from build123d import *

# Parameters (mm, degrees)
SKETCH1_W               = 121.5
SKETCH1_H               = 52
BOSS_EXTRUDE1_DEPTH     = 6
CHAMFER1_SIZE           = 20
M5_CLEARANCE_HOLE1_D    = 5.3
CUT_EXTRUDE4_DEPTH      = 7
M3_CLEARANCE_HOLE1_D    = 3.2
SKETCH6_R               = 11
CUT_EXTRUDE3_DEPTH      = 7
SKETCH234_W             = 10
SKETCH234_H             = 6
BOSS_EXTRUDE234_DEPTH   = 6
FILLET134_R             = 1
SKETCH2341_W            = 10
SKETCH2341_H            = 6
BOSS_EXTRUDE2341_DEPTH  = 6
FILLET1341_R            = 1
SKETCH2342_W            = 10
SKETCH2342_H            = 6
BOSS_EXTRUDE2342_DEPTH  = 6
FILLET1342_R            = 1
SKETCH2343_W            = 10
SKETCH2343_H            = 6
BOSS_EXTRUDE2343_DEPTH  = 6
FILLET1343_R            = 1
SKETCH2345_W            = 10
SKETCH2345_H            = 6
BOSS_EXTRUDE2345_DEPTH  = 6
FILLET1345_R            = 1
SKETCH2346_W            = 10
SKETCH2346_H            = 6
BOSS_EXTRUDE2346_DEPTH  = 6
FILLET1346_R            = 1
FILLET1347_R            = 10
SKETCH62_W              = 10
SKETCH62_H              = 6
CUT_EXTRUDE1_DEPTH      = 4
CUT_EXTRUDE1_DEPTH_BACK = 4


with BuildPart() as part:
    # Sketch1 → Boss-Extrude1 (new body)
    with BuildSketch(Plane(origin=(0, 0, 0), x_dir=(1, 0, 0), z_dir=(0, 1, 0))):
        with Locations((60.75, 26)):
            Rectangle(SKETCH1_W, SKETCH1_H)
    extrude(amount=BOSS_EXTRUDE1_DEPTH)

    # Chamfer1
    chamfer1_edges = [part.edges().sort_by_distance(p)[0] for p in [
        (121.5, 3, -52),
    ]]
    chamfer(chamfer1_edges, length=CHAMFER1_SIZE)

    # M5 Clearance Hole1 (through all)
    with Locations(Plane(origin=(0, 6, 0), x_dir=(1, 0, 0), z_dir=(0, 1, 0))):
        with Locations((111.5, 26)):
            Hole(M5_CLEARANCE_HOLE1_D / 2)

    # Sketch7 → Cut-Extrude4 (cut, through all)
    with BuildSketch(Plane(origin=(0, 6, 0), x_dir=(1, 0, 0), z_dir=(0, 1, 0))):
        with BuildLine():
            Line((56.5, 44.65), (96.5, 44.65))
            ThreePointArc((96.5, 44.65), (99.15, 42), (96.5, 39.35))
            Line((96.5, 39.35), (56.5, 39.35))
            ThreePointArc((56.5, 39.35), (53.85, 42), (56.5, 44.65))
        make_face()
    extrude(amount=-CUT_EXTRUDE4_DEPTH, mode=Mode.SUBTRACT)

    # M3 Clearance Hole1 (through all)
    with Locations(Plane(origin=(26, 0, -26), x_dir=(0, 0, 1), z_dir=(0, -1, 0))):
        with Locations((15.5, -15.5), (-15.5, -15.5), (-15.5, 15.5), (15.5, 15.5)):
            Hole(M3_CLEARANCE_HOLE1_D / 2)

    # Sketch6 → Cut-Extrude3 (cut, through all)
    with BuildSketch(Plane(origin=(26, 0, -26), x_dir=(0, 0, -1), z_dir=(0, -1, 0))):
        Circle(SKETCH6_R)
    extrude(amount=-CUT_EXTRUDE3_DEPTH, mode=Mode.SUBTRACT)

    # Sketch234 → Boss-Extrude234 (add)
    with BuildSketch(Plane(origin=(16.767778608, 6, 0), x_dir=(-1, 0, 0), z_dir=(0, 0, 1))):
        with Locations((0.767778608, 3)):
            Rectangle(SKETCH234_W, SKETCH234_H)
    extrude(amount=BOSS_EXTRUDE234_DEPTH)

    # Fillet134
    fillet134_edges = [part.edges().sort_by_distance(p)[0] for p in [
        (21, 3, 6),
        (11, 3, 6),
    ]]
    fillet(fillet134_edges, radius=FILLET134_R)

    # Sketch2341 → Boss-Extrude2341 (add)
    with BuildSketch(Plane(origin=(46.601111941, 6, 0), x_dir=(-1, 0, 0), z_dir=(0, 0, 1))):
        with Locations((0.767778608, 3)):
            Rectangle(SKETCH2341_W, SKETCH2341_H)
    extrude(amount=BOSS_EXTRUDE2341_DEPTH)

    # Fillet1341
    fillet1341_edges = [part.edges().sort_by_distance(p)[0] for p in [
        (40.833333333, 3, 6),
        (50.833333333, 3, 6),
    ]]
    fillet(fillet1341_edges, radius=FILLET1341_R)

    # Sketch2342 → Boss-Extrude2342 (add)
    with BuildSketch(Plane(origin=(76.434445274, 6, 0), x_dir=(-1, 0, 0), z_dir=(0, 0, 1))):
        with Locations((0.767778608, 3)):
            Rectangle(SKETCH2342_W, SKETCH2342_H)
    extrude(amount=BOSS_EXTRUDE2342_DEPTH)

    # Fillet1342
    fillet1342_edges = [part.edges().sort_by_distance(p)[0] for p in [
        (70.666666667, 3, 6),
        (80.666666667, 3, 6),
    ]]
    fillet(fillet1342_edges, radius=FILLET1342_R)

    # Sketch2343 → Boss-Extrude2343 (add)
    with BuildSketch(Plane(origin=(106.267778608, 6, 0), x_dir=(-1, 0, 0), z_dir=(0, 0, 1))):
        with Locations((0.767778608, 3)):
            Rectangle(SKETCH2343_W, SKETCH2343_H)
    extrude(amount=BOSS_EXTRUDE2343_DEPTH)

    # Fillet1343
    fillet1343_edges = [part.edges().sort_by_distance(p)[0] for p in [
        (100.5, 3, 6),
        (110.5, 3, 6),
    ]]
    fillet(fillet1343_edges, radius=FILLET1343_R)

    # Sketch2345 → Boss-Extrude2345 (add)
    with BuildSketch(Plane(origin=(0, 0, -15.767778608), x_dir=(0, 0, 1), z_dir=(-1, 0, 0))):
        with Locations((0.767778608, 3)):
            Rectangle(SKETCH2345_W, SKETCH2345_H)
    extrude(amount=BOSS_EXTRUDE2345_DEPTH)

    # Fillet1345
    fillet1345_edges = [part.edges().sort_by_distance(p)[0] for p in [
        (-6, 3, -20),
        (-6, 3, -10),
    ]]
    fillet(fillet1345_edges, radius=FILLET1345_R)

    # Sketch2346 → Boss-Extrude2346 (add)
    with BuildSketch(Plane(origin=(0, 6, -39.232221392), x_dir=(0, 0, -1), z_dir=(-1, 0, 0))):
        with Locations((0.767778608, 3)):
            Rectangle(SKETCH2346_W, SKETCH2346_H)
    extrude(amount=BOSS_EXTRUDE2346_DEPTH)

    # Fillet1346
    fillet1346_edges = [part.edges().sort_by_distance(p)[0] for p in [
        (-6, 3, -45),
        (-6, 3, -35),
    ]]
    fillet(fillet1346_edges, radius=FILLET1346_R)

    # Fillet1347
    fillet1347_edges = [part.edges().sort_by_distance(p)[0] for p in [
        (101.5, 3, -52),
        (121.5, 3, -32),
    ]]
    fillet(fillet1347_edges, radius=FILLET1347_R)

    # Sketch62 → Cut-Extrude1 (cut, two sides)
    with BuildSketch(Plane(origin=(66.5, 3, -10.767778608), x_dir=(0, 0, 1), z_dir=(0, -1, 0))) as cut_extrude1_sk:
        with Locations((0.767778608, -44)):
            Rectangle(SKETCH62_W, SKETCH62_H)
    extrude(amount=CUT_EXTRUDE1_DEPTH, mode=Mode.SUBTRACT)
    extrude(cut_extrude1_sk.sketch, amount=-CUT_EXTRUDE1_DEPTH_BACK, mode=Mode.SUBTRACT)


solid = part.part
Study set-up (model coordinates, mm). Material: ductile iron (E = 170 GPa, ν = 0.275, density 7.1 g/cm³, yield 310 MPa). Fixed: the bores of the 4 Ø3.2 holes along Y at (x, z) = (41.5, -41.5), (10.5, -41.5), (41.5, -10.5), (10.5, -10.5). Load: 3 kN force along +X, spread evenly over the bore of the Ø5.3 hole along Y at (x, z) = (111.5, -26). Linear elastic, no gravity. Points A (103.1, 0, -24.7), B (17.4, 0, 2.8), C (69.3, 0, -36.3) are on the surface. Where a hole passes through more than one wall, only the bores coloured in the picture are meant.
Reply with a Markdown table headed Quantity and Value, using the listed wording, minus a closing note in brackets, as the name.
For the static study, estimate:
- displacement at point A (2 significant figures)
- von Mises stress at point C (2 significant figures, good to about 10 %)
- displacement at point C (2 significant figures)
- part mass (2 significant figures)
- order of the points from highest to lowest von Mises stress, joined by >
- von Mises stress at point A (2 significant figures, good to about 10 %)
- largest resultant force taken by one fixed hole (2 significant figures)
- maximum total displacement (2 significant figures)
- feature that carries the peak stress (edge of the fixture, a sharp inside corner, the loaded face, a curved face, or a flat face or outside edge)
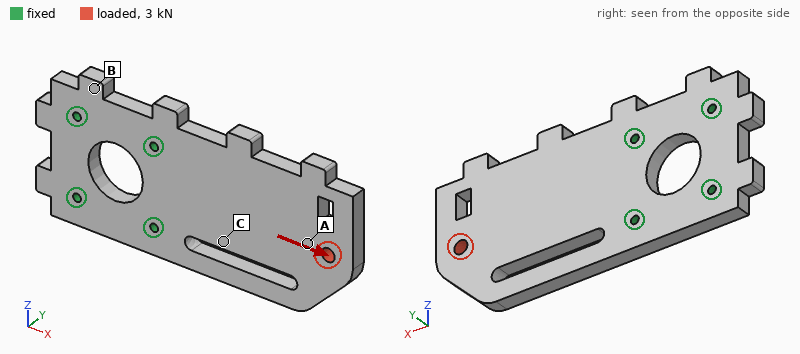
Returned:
| Quantity | Value |
|---|---|
| displacement at point A | 6.0 µm |
| von Mises stress at point C | 15 MPa |
| displacement at point C | 2.9 µm |
| part mass | 240 g |
| order of the points from highest to lowest von Mises stress, joined by > | A > C > B |
| von Mises stress at point A | 25 MPa |
| largest resultant force taken by one fixed hole | 1.4 kN |
| maximum total displacement | 8.0 µm |
| feature that carries the peak stress | the loaded face |
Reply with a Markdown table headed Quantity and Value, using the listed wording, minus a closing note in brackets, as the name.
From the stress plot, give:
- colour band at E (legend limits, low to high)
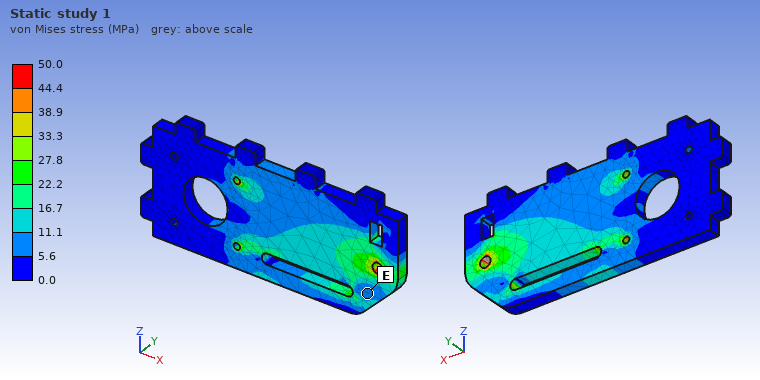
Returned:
| Quantity | Value |
|---|---|
| colour band at E | 5.6 to 11.1 MPa |
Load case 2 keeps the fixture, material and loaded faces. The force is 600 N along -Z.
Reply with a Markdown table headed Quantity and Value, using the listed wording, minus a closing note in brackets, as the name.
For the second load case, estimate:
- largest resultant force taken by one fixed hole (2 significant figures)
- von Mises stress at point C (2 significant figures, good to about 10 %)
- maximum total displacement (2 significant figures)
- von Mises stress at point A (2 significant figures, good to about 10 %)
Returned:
| Quantity | Value |
|---|---|
| largest resultant force taken by one fixed hole | 1.1 kN |
| von Mises stress at point C | 8.1 MPa |
| maximum total displacement | 15 µm |
| von Mises stress at point A | 4.4 MPa |
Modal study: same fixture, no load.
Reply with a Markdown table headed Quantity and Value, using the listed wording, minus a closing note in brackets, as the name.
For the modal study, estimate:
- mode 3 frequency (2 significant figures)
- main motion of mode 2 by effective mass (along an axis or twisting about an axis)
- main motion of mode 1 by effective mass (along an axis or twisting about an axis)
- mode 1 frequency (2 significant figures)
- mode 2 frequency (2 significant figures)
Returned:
| Quantity | Value |
|---|---|
| mode 3 frequency | 4400 Hz |
| main motion of mode 2 by effective mass | twisting about X |
| main motion of mode 1 by effective mass | along Y |
| mode 1 frequency | 760 Hz |
| mode 2 frequency | 2500 Hz |
